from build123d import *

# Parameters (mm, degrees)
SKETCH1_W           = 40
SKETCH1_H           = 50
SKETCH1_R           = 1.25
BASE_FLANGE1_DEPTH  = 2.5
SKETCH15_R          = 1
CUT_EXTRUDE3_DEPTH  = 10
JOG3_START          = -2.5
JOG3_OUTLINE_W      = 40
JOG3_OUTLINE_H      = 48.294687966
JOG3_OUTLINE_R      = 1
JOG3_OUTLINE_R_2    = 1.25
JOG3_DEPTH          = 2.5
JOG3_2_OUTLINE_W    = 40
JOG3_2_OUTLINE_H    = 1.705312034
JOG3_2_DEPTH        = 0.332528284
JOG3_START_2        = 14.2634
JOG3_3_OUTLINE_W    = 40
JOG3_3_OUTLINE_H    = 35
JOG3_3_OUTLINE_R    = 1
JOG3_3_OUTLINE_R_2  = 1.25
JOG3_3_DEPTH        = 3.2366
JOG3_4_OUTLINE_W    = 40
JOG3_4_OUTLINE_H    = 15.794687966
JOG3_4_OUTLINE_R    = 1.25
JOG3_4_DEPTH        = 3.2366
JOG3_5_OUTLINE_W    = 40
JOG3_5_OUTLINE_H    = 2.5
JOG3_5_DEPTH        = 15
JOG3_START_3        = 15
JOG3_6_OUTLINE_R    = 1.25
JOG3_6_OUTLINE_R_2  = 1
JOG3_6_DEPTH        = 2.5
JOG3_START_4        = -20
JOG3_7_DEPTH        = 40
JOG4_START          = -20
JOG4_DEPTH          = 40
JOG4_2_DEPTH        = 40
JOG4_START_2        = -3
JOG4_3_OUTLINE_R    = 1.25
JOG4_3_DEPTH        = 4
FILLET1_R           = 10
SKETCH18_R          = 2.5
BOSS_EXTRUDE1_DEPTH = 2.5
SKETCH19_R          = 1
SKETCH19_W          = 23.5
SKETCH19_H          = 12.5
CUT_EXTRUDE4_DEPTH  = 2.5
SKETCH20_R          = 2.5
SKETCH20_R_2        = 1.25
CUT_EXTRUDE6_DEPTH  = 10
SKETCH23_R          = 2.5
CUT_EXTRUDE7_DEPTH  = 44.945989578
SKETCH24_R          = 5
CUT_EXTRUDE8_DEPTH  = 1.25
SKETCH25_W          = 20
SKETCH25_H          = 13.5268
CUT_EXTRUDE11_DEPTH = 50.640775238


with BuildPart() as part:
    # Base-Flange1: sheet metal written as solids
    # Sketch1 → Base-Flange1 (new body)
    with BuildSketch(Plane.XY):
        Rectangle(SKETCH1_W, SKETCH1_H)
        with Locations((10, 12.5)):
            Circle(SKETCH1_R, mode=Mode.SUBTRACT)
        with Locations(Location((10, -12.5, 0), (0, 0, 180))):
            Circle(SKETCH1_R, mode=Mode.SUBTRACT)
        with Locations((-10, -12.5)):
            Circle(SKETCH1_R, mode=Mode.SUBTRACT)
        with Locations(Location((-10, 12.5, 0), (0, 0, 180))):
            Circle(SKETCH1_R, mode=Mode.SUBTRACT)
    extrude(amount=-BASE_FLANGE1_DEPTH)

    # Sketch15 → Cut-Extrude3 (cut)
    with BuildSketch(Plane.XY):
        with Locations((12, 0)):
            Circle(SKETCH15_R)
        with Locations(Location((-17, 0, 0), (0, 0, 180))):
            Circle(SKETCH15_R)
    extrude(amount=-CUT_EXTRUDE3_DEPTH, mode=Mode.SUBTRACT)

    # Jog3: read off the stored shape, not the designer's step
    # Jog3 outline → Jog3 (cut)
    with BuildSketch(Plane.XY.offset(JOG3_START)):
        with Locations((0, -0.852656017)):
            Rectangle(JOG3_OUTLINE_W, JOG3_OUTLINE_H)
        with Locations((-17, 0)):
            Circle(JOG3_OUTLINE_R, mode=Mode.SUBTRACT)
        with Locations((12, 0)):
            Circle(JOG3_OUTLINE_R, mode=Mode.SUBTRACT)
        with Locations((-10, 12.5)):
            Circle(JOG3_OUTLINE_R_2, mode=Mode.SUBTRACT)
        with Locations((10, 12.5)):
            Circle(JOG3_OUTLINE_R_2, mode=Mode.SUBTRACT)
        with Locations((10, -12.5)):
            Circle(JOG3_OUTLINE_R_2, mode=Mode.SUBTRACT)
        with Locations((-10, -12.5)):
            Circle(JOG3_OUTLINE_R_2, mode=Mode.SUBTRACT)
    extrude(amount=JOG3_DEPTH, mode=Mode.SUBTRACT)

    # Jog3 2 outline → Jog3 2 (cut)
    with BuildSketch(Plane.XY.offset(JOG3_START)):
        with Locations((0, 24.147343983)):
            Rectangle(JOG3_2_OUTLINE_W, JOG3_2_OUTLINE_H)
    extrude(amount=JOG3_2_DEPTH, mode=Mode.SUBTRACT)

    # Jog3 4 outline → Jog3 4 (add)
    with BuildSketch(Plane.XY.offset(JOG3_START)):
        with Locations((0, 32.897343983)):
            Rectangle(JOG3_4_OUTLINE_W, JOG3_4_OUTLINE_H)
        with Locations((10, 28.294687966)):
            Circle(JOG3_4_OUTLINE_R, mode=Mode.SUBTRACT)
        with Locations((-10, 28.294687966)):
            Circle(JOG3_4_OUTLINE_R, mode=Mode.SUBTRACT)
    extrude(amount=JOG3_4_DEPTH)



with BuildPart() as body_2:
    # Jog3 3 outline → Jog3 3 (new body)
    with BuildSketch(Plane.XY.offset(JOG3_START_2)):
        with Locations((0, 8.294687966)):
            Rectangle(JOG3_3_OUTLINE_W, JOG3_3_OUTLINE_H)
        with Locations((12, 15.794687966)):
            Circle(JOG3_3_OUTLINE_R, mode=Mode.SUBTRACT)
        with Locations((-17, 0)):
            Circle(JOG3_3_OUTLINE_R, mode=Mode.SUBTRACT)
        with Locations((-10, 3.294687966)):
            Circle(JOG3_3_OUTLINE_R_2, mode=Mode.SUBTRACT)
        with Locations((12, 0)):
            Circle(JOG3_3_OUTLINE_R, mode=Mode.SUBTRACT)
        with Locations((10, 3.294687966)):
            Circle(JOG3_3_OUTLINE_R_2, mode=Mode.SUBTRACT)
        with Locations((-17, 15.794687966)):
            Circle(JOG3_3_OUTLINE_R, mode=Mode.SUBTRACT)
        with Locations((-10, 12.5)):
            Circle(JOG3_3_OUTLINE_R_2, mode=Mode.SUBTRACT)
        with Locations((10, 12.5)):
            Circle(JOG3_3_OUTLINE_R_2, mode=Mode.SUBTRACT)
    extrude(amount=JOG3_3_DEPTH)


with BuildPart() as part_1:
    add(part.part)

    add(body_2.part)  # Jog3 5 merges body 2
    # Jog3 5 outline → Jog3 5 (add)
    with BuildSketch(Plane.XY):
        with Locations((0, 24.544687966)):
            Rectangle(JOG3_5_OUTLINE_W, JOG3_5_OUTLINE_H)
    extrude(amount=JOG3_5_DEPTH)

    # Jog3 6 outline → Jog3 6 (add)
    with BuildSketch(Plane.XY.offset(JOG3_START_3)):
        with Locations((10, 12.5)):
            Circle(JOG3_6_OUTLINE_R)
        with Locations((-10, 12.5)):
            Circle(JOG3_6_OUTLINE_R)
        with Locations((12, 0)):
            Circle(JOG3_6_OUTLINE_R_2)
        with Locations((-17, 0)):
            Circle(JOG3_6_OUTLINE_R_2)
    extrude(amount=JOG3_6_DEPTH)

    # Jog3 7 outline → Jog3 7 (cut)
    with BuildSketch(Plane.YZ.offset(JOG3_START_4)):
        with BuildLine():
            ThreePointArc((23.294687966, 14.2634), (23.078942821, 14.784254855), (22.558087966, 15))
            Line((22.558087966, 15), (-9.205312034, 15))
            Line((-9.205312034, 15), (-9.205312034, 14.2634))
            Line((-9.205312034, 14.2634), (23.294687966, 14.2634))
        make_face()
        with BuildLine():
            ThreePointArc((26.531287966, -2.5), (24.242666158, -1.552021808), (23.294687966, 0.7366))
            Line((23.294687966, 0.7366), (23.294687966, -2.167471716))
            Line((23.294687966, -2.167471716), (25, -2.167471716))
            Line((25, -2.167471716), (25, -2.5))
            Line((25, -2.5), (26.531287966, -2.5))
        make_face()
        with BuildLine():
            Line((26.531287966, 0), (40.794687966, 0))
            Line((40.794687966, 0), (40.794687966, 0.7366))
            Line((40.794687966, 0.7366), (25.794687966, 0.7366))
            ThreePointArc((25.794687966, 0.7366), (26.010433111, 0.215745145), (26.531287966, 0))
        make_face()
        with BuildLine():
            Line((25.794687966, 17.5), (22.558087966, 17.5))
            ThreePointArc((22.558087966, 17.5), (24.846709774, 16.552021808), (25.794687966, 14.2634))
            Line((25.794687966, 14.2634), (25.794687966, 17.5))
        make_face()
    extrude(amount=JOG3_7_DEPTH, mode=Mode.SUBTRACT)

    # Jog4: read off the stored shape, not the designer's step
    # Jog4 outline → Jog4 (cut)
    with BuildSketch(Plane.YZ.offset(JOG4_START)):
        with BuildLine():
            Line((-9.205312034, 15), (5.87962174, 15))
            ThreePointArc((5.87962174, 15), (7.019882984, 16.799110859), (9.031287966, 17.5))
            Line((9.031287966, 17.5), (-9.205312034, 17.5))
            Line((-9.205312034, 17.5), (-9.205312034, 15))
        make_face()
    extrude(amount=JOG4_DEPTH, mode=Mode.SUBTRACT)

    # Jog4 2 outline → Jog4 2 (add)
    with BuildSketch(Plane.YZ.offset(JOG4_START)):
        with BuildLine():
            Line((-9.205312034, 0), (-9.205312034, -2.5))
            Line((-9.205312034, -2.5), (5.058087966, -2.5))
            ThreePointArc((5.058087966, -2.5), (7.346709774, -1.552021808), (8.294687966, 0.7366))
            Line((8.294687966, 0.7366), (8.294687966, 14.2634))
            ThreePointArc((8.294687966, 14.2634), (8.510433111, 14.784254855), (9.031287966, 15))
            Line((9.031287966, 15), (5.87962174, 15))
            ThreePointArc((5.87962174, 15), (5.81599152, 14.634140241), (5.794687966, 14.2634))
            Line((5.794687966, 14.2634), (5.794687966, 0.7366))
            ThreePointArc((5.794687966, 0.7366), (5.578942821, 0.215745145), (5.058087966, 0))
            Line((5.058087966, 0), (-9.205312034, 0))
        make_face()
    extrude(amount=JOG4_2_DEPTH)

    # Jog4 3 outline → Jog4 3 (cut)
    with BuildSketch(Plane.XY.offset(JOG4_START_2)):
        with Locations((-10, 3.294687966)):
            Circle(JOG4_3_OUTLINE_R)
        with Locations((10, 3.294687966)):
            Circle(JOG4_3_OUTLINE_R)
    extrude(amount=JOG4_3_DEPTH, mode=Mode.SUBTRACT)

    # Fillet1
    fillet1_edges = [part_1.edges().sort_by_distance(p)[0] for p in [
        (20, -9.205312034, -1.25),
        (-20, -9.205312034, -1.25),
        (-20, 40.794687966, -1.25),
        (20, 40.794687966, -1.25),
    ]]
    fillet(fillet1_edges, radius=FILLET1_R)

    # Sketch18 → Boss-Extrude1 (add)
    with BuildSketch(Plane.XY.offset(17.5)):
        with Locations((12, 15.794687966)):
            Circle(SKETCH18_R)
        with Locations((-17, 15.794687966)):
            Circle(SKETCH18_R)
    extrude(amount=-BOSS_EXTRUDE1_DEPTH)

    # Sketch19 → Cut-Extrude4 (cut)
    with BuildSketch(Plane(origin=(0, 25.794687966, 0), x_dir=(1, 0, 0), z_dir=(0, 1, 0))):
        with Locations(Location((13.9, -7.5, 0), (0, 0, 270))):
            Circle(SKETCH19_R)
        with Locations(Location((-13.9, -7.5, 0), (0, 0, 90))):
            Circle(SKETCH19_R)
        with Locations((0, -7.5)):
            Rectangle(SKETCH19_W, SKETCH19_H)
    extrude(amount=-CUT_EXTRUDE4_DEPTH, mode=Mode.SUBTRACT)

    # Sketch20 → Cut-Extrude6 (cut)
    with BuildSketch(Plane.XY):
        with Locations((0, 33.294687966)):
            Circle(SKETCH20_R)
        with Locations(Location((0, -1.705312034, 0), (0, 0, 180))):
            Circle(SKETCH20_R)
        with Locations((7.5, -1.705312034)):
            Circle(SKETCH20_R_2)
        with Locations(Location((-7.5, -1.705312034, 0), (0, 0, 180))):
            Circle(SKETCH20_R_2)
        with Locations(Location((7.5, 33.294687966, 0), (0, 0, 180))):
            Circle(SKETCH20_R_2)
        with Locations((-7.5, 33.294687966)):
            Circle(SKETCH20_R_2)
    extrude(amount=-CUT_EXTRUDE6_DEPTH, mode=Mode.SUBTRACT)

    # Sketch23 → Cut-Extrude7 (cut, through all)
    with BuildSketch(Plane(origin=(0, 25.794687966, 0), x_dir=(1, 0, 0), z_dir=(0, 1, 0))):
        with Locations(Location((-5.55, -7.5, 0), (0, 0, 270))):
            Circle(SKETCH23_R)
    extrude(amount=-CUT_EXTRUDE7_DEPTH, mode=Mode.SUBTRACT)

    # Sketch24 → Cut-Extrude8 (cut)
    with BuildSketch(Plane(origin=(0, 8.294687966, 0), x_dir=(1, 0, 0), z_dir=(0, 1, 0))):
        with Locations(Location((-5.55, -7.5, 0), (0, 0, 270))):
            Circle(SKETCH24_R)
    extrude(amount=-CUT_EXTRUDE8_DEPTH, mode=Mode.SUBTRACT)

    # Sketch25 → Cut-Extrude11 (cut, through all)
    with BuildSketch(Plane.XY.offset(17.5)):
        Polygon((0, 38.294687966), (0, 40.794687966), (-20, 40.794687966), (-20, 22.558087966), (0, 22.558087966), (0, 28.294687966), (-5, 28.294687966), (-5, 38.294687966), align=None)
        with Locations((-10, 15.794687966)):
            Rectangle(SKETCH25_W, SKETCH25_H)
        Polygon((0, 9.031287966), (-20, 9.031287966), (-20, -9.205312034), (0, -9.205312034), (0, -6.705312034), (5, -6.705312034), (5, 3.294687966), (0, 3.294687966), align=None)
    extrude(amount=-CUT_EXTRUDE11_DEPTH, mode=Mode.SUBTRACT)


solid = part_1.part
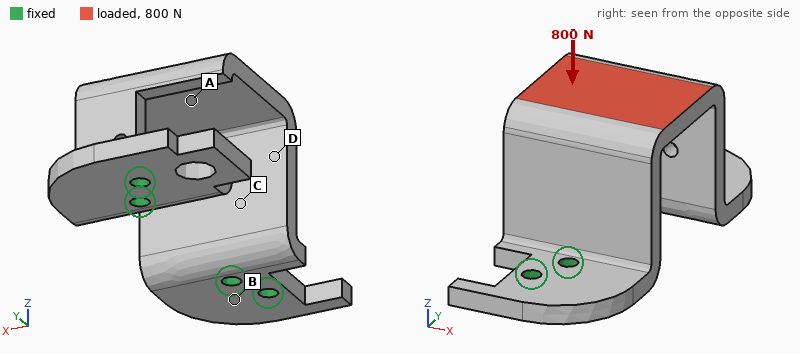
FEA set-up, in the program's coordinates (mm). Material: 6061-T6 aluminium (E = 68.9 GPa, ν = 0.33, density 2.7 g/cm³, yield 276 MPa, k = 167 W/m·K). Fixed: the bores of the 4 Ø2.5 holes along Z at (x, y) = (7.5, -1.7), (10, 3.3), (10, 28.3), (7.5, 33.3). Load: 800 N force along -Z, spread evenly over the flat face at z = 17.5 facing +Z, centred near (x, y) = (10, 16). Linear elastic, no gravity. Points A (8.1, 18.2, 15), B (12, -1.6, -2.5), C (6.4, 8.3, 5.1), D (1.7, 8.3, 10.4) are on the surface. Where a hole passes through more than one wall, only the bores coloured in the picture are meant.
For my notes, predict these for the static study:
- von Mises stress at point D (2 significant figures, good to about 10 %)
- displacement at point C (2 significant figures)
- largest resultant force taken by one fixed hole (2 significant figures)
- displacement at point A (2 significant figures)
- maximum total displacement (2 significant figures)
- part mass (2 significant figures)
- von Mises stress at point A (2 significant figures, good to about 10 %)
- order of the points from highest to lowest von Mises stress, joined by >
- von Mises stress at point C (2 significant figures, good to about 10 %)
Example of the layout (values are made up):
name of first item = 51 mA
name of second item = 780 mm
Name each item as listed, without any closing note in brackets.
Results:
von Mises stress at point D = 45 MPa
displacement at point C = 0.021 mm
largest resultant force taken by one fixed hole = 430 N
displacement at point A = 0.064 mm
maximum total displacement = 0.11 mm
part mass = 9.4 g
von Mises stress at point A = 63 MPa
order of the points from highest to lowest von Mises stress, joined by > = A > D > C > B
von Mises stress at point C = 22 MPa
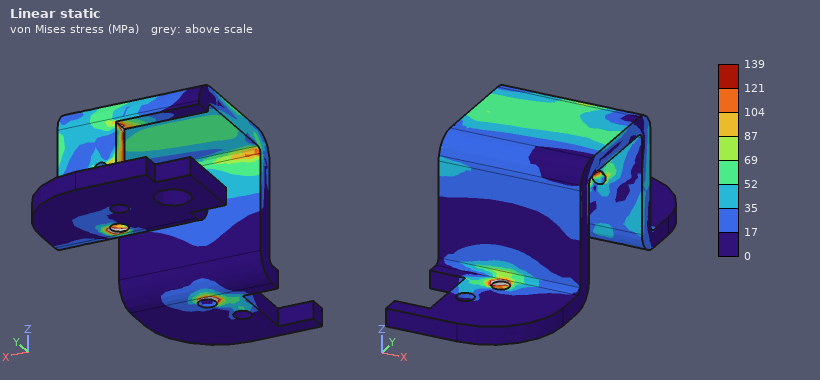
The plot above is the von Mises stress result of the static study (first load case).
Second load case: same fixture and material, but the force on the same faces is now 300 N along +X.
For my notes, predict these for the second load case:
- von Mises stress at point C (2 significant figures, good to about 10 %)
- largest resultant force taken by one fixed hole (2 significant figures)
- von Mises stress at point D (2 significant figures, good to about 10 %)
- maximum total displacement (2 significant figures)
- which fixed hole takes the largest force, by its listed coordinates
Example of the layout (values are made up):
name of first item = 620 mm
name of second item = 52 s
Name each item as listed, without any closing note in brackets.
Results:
von Mises stress at point C = 21 MPa
largest resultant force taken by one fixed hole = 330 N
von Mises stress at point D = 21 MPa
maximum total displacement = 0.16 mm
which fixed hole takes the largest force, by its listed coordinates = (10, 3.3)
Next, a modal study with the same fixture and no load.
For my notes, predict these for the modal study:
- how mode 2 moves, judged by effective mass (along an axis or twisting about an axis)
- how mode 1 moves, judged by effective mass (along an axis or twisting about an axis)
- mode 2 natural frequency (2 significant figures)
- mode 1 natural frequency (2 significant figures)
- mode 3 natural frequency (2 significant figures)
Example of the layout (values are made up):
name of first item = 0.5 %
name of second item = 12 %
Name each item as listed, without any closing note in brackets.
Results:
how mode 2 moves, judged by effective mass = along Y
how mode 1 moves, judged by effective mass = along X
mode 2 natural frequency = 4800 Hz
mode 1 natural frequency = 4100 Hz
mode 3 natural frequency = 7300 Hz
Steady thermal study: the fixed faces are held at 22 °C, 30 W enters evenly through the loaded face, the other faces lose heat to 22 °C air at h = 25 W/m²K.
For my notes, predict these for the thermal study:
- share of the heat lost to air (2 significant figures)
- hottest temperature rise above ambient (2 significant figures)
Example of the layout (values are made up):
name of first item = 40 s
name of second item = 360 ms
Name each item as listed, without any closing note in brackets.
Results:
share of the heat lost to air = 6.4 %
hottest temperature rise above ambient = 70 K
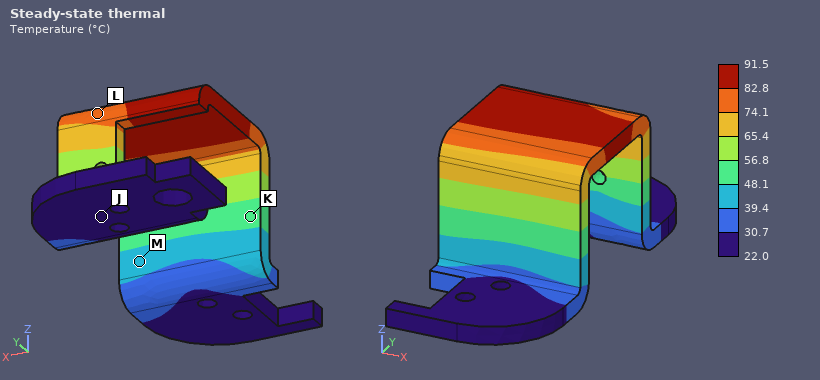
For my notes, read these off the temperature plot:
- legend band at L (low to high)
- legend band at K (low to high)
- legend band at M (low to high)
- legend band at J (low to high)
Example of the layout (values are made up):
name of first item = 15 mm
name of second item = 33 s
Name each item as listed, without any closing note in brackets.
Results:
legend band at L = 74.1 to 82.8 °C
legend band at K = 48.1 to 56.8 °C
legend band at M = 39.4 to 48.1 °C
legend band at J = 22.0 to 30.7 °C
